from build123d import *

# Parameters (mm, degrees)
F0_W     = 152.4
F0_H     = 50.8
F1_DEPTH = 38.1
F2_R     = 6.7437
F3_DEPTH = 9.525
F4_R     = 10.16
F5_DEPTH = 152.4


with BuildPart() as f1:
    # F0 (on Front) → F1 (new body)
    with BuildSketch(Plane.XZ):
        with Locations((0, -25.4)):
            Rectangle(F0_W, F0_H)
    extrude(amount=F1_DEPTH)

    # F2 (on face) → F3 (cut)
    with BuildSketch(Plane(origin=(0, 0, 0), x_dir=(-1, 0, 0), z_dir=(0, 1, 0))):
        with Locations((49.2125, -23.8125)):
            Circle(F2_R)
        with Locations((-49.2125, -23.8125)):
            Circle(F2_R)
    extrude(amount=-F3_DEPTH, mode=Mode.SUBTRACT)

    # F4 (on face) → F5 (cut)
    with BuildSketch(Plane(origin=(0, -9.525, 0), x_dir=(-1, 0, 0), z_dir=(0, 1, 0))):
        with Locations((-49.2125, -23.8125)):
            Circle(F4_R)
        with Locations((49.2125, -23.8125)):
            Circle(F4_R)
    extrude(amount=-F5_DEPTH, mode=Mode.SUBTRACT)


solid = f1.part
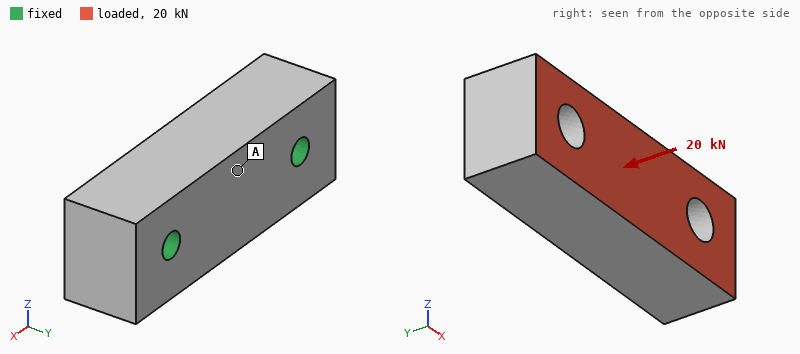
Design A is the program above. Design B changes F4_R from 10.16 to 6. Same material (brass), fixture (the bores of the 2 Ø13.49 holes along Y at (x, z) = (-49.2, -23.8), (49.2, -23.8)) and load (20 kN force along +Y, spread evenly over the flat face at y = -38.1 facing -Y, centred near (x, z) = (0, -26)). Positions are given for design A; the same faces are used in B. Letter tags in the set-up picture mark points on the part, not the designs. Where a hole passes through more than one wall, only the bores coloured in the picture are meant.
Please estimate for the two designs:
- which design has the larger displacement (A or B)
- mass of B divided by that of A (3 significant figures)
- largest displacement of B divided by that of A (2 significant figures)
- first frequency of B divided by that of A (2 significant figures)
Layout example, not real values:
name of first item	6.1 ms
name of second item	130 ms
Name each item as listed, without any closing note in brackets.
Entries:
which design has the larger displacement	A
mass of B divided by that of A	1.04
largest displacement of B divided by that of A	0.73
first frequency of B divided by that of A	1.2
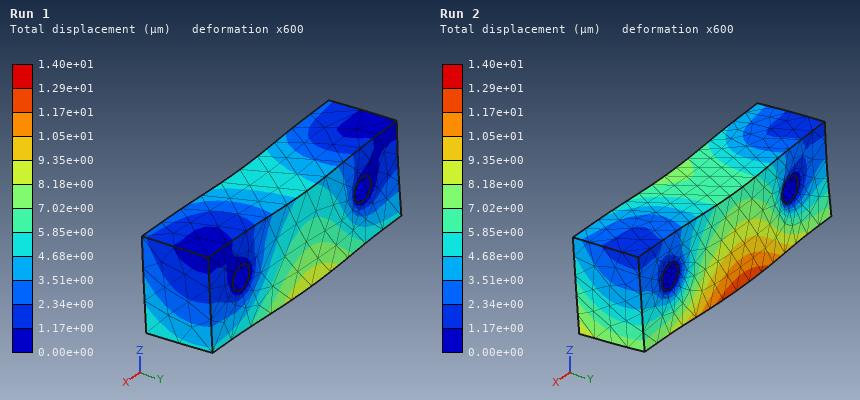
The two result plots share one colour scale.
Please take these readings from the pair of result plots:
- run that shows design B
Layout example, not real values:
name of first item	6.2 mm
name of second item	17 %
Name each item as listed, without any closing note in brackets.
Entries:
run that shows design B	Run 1
